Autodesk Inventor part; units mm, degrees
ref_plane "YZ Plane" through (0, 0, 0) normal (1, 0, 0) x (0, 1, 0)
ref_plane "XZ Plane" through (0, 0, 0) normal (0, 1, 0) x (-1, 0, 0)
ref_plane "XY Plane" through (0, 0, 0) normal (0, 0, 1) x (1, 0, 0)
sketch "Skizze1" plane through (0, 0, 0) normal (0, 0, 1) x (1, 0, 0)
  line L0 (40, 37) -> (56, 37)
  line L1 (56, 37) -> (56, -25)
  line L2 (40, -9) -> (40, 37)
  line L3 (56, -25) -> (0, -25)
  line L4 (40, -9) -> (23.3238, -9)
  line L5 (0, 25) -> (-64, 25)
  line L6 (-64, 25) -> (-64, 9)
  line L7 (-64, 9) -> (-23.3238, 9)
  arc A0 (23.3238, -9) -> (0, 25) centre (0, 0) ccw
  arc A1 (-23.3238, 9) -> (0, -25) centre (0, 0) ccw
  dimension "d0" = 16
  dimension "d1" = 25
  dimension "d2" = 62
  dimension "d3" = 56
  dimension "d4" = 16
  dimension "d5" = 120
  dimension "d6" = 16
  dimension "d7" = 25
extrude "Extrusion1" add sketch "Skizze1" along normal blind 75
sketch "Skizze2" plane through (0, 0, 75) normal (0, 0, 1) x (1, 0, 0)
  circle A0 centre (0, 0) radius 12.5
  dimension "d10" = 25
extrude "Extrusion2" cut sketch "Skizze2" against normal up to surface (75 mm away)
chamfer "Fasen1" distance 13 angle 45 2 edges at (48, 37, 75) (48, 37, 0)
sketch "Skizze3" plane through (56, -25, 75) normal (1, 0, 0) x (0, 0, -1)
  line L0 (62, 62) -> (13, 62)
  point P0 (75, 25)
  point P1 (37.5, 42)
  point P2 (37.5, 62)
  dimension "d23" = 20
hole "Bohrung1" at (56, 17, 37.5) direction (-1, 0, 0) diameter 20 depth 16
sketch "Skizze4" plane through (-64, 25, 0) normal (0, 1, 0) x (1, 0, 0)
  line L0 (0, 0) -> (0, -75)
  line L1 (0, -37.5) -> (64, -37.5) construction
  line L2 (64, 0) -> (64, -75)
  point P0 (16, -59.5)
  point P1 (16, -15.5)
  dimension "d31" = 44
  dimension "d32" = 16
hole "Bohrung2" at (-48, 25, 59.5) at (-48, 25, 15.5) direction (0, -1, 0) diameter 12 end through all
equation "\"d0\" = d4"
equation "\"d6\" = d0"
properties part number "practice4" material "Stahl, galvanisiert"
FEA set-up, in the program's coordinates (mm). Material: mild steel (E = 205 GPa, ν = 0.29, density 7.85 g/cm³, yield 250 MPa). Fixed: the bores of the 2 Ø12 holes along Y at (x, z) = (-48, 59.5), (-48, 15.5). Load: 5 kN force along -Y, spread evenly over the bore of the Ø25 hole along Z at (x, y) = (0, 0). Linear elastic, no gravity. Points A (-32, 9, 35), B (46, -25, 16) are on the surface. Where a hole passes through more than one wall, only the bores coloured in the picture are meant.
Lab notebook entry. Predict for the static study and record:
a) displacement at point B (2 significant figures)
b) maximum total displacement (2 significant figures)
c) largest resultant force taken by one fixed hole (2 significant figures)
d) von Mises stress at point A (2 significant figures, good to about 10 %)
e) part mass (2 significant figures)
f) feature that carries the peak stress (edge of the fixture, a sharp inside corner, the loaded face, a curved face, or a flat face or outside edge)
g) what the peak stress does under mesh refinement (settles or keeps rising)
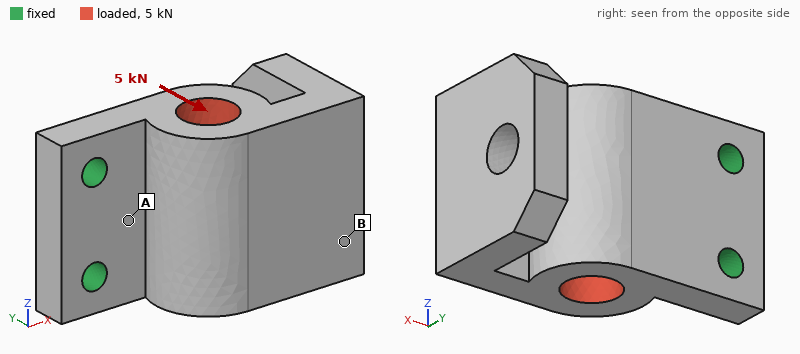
87 µm
95 µm
2.5 kN
38 MPa
2.0 kg
edge of the fixture
keeps rising
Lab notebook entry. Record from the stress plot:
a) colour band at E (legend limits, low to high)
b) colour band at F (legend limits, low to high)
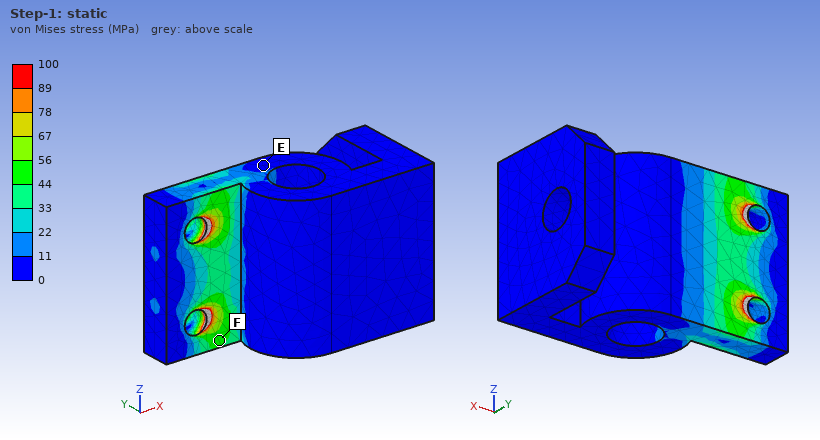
0 to 11 MPa
44 to 56 MPa
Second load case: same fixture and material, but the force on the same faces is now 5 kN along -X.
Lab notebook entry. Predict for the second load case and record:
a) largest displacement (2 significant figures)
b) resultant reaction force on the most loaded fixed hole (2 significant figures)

50 µm
2.5 kN
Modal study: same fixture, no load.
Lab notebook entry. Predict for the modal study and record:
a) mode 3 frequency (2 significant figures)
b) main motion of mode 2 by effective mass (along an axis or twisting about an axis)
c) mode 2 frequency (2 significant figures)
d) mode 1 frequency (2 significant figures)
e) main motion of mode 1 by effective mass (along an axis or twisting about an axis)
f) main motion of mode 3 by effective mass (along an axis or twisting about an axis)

2600 Hz
along Z
2300 Hz
800 Hz
along Y
along X
